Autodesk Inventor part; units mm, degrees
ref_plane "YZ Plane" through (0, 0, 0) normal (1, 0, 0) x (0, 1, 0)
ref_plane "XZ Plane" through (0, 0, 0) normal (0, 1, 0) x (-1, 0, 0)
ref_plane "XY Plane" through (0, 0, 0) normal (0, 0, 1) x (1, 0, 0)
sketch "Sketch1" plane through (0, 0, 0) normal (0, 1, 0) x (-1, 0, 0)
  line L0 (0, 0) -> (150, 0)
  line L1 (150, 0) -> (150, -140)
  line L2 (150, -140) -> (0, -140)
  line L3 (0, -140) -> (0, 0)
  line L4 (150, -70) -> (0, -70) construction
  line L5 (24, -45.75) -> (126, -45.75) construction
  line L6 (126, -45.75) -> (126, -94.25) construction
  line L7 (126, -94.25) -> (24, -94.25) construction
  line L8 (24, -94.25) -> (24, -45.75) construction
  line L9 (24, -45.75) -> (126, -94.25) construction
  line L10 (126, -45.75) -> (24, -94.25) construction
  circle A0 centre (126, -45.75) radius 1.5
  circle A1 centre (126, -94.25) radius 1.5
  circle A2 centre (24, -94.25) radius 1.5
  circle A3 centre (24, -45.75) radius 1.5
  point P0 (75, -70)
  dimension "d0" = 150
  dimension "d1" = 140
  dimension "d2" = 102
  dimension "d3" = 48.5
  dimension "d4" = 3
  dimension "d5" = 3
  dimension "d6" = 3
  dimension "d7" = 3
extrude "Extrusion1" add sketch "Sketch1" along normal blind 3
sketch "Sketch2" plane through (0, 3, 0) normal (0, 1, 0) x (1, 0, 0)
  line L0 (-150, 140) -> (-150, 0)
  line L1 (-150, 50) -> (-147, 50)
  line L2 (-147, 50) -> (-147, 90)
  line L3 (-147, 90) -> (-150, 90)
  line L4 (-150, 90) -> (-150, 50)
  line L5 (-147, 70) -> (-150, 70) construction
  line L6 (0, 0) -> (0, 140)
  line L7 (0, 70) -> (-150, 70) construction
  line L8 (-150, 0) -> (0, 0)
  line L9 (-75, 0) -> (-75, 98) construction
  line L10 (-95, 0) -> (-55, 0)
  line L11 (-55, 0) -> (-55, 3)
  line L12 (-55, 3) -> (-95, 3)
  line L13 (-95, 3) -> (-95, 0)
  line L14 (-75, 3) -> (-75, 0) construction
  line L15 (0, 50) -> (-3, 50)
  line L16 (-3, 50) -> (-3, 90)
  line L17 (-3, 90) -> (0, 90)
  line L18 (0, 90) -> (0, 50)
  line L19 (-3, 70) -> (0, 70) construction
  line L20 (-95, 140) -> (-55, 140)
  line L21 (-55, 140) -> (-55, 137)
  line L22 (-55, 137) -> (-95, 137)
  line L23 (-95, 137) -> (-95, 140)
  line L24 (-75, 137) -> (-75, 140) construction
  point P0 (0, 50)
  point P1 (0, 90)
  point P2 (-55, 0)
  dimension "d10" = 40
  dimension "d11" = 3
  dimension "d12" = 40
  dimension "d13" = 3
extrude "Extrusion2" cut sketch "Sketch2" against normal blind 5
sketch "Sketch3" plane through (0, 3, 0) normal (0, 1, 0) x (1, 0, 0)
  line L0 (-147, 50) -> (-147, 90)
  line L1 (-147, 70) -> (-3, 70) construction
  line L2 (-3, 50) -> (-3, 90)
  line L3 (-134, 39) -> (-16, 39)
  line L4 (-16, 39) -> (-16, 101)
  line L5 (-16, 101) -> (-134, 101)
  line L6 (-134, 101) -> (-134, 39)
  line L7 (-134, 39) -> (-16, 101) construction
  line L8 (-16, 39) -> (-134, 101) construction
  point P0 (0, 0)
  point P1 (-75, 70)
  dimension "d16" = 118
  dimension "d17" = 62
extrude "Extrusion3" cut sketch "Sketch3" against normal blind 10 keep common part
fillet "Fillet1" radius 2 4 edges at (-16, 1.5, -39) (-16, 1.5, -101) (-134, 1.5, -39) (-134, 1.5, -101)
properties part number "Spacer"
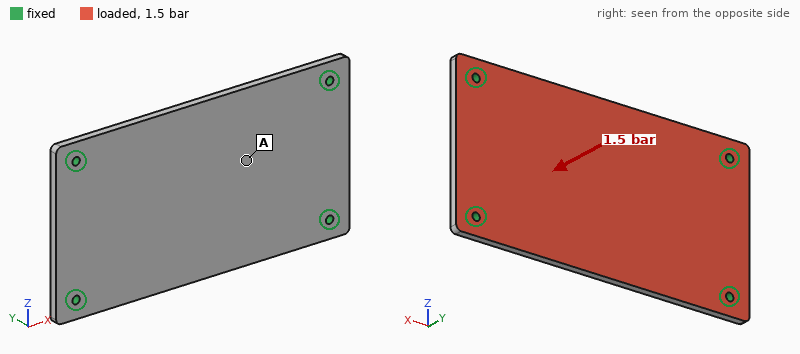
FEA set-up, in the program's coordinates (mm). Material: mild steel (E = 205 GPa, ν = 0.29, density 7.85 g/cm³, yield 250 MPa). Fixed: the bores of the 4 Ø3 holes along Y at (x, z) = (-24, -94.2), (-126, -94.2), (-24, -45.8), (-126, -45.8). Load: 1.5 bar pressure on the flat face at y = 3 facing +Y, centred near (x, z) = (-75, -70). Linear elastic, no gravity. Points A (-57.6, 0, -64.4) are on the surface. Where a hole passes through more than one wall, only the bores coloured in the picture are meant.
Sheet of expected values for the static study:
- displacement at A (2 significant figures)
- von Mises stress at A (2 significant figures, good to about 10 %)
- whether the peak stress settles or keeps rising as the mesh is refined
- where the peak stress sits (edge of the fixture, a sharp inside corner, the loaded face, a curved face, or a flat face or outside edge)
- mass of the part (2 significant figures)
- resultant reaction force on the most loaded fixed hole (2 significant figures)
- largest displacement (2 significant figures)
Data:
0.098 mm
30 MPa
keeps rising
edge of the fixture
170 g
270 N
0.12 mm
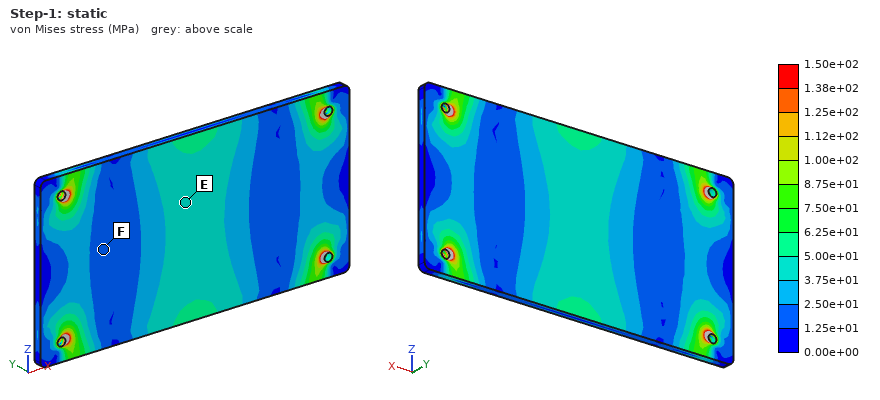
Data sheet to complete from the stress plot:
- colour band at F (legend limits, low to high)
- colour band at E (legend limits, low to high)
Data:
1.25e+01 to 2.50e+01 MPa
3.75e+01 to 5.00e+01 MPa
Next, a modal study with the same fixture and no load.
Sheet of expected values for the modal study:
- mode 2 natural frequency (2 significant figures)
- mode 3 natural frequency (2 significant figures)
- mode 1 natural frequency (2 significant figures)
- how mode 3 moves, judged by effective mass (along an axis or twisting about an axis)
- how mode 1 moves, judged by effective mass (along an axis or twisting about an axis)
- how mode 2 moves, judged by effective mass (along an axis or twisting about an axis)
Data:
2200 Hz
3600 Hz
1300 Hz
twisting about Z
along Y
twisting about X
